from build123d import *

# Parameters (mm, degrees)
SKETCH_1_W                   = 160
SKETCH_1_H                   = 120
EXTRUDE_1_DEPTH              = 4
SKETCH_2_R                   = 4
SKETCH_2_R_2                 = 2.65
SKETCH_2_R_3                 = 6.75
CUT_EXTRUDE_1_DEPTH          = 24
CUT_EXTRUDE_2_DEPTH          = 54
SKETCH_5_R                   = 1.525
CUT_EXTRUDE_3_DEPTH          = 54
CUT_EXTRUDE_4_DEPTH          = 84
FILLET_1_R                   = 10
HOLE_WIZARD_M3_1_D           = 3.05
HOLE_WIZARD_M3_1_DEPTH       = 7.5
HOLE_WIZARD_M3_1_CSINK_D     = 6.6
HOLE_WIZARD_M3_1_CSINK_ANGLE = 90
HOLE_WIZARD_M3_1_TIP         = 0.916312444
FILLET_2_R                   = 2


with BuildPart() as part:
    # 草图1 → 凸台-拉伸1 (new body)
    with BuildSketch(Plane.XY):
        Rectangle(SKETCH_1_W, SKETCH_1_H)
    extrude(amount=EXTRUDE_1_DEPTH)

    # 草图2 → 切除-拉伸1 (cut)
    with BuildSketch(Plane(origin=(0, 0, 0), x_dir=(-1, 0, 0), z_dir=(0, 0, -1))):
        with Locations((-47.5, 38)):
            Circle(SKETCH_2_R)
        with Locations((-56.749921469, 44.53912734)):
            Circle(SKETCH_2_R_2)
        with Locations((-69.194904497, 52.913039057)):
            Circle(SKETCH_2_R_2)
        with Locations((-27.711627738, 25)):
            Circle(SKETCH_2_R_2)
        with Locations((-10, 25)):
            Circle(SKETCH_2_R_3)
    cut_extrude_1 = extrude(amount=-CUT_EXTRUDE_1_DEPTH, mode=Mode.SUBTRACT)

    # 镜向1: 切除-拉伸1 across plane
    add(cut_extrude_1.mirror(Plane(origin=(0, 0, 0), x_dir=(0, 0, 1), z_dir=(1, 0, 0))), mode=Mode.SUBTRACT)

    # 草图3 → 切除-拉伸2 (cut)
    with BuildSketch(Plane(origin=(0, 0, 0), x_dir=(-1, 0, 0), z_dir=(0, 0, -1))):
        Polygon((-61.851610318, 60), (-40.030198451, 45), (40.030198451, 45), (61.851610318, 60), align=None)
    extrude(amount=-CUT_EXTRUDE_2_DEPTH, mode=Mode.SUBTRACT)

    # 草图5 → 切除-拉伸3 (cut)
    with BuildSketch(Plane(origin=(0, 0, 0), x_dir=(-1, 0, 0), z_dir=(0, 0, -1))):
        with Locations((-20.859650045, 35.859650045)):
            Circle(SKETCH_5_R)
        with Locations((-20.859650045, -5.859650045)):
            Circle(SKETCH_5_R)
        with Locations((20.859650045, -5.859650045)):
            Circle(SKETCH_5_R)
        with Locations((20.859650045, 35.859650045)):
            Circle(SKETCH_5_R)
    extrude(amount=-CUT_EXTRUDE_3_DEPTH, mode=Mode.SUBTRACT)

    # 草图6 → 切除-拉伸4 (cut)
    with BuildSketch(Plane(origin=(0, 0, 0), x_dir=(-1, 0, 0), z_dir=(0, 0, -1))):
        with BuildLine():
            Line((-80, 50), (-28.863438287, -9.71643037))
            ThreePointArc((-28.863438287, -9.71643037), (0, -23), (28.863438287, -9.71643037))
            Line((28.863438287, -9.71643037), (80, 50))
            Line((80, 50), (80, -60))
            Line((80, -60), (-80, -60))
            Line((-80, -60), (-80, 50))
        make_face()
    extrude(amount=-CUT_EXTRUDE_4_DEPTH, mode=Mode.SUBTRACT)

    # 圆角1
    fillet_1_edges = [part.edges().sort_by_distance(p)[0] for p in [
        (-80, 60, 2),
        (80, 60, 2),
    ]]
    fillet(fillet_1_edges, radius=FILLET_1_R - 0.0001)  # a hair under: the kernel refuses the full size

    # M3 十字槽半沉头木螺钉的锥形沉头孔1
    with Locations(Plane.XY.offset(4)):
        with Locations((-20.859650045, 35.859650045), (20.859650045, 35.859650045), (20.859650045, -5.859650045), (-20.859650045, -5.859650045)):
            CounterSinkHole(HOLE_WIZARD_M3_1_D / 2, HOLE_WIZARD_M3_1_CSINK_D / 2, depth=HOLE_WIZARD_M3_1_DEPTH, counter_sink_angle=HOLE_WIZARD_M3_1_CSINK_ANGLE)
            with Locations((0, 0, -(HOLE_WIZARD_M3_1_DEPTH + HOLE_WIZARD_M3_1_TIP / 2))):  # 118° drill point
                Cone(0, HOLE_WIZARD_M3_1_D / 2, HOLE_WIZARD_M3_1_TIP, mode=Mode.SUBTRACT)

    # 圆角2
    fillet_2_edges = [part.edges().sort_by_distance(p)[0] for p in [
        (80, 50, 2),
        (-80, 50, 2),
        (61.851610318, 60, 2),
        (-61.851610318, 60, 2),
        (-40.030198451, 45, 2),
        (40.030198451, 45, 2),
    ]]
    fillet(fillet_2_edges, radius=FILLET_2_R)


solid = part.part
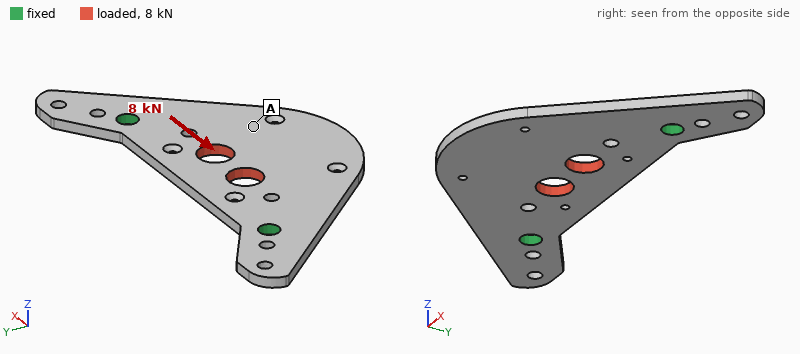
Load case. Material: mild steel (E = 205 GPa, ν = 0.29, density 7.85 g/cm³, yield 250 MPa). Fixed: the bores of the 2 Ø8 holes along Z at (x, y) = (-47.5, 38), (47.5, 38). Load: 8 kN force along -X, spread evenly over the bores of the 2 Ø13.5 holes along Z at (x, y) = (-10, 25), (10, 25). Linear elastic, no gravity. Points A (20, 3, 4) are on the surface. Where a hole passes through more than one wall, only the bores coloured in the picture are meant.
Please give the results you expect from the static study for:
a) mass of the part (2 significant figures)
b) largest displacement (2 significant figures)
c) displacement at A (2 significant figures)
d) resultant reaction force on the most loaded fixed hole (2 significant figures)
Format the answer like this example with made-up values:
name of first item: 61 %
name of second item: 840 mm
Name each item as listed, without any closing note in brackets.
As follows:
mass of the part: 200 g
largest displacement: 13 µm
displacement at A: 8.8 µm
resultant reaction force on the most loaded fixed hole: 4.1 kN
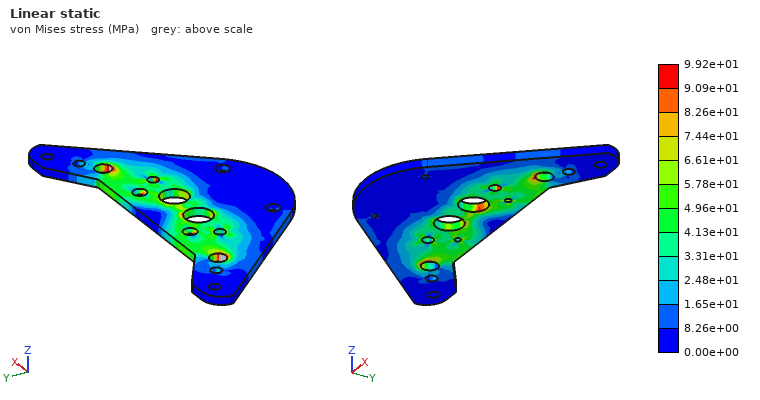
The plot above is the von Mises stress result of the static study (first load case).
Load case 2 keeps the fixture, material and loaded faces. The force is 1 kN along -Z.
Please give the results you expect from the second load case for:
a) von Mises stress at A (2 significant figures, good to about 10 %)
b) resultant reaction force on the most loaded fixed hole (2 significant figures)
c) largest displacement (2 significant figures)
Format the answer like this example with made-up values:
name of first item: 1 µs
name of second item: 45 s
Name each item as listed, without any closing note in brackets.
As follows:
von Mises stress at A: 39 MPa
resultant reaction force on the most loaded fixed hole: 500 N
largest displacement: 0.17 mm
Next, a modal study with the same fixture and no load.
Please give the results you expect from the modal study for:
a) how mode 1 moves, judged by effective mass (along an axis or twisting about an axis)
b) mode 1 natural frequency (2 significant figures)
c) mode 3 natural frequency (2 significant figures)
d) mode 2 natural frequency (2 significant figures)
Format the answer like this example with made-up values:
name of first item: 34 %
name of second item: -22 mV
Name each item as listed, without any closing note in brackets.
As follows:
how mode 1 moves, judged by effective mass: along Z
mode 1 natural frequency: 900 Hz
mode 3 natural frequency: 2800 Hz
mode 2 natural frequency: 2800 Hz
